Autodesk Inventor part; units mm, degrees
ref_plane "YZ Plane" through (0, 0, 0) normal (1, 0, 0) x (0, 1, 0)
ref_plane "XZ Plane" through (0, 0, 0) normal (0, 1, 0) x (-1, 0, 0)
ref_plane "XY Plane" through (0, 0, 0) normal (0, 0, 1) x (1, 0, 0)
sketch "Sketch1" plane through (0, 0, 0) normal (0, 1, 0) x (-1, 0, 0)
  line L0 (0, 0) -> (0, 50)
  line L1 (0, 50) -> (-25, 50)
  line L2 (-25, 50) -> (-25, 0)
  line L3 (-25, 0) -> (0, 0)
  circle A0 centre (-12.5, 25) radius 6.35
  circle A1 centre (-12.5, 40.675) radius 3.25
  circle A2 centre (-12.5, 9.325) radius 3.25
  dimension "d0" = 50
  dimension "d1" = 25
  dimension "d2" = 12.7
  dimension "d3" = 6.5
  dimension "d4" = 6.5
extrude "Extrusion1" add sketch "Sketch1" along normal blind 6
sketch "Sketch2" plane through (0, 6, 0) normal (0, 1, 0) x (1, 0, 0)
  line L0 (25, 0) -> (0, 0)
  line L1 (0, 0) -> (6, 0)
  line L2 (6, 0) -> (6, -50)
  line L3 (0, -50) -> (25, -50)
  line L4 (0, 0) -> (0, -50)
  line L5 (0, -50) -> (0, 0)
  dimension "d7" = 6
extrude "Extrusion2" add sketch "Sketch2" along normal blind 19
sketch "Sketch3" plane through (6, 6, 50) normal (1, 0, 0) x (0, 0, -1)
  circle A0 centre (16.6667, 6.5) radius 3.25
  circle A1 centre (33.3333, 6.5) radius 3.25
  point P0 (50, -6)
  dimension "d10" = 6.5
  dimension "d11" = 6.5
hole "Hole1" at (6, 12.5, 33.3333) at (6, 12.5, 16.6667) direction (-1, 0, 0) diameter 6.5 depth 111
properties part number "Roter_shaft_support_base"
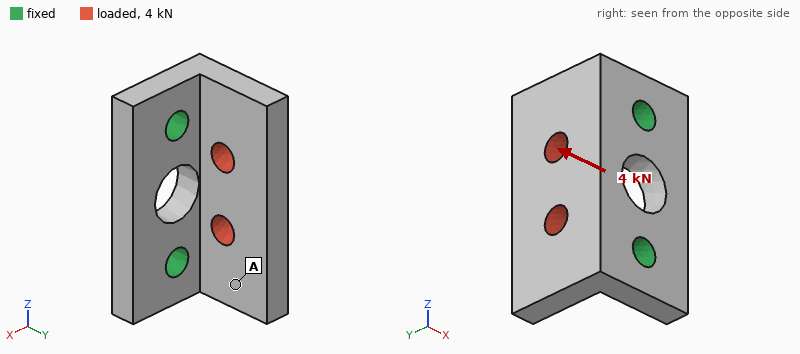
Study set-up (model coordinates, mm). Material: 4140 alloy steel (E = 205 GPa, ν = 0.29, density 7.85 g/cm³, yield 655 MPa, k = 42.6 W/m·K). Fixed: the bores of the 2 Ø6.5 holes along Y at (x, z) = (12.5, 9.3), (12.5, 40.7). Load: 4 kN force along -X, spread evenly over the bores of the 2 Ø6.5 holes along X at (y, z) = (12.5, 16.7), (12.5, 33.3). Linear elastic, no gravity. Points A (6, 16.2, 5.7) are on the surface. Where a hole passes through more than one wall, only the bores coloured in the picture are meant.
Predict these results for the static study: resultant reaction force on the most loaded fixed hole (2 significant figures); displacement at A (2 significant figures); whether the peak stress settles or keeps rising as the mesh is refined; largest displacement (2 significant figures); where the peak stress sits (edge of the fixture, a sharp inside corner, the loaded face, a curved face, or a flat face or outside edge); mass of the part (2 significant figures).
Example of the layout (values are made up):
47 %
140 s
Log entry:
2.1 kN
30 µm
keeps rising
66 µm
edge of the fixture
91 g
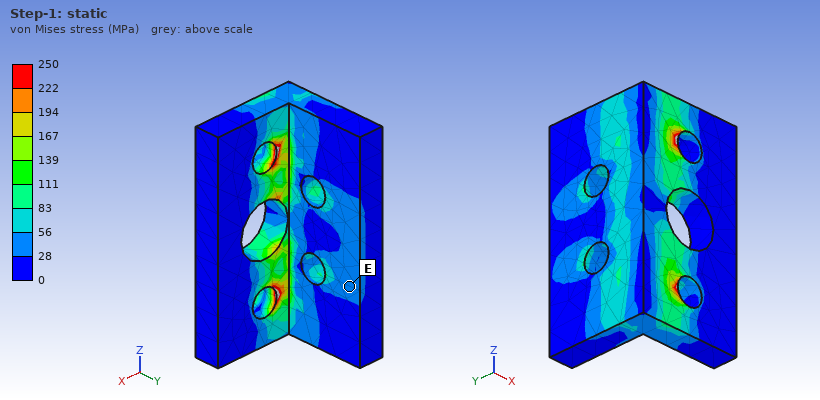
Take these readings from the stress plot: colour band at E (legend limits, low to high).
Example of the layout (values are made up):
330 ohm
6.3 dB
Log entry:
28 to 56 MPa
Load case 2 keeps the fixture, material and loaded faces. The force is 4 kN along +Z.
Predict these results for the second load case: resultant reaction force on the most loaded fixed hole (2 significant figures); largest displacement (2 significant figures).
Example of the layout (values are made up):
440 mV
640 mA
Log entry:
2.4 kN
11 µm
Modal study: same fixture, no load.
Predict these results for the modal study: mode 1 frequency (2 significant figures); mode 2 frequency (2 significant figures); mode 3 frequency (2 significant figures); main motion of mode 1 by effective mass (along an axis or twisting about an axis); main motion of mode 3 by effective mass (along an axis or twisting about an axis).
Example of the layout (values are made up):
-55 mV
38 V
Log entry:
6100 Hz
10 kHz
16 kHz
along X
along Z
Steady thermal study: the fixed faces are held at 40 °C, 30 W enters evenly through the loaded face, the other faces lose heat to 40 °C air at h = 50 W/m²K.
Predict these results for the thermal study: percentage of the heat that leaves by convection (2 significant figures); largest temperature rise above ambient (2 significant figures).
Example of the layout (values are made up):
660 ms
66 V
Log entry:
17 %
50 K
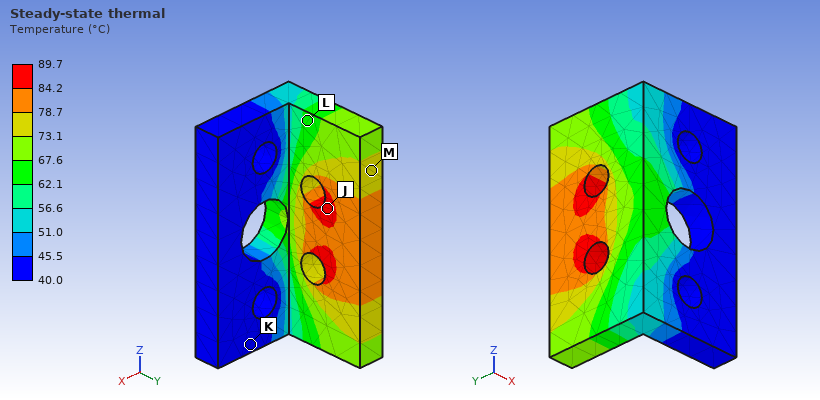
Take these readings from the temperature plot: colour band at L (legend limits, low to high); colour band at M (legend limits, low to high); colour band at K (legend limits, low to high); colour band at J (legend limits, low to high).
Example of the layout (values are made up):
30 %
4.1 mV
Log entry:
62.1 to 67.6 °C
73.1 to 78.7 °C
40.0 to 45.5 °C
84.2 to 89.7 °C
